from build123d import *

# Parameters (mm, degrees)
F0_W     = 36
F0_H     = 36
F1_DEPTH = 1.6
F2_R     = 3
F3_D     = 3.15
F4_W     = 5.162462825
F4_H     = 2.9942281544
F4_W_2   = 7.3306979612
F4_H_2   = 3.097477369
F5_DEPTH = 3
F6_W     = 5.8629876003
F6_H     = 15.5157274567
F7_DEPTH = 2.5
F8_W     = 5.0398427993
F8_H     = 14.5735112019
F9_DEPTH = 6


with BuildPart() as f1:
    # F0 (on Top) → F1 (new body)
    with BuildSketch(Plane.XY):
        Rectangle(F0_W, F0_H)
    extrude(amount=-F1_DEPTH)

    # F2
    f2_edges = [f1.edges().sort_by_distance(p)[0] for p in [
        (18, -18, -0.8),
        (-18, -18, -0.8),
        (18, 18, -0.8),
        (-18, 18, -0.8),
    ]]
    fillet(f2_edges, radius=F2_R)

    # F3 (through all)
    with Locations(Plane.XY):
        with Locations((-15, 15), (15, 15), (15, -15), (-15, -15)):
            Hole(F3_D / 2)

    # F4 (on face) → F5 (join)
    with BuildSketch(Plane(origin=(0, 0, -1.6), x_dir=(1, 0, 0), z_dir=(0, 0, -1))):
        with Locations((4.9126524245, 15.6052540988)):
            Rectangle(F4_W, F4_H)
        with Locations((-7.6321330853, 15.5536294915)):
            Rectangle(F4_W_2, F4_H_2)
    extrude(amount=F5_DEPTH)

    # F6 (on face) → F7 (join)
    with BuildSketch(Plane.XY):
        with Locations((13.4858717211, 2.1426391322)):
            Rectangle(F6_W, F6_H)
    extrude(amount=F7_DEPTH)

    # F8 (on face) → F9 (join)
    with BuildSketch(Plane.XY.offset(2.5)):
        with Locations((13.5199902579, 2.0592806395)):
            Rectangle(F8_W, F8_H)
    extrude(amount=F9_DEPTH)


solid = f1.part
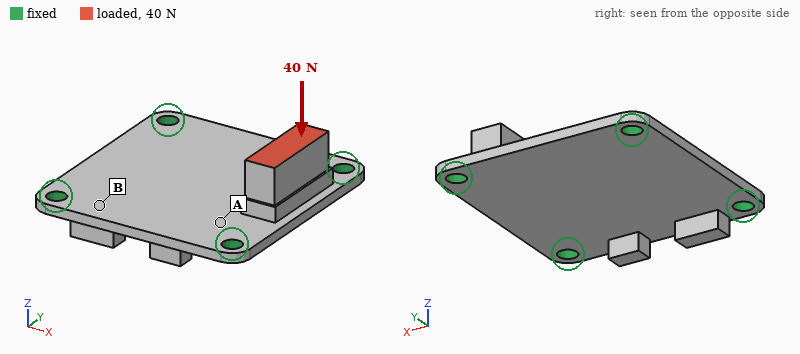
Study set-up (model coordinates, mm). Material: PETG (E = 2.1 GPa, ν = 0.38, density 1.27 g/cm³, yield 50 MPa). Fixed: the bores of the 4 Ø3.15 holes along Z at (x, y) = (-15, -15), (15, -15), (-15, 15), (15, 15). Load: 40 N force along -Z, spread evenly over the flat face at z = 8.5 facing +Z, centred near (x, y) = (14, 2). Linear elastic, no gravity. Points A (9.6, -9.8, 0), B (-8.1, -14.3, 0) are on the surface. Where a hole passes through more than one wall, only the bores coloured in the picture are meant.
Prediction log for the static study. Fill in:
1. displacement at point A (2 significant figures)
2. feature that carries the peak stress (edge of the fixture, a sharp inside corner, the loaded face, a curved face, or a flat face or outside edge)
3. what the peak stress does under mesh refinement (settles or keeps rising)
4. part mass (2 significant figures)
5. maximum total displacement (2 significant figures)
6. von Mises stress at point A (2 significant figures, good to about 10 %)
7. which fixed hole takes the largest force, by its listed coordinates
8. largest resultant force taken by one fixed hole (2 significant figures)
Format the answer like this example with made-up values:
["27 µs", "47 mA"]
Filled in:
["0.076 mm", "edge of the fixture", "keeps rising", "3.5 g", "0.16 mm", "3.5 MPa", "(15, 15)", "24 N"]
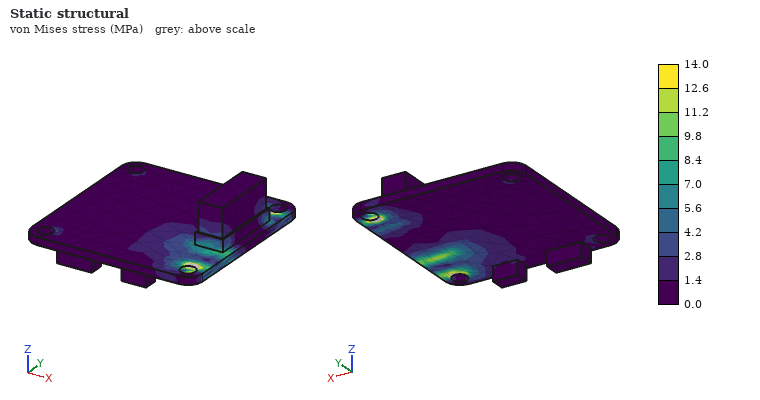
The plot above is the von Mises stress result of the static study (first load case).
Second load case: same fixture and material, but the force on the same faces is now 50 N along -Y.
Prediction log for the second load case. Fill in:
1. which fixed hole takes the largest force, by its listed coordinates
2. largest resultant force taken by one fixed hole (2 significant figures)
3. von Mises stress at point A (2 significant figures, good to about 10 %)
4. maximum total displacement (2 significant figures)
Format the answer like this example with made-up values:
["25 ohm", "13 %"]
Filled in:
["(15, 15)", "31 N", "4.7 MPa", "0.20 mm"]
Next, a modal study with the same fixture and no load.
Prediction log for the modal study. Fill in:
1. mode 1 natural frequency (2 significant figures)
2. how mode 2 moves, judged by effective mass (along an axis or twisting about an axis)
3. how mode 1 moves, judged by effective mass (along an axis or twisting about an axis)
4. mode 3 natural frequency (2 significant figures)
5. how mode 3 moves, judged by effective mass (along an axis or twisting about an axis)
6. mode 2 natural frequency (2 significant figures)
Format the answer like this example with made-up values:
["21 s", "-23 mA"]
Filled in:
["1700 Hz", "along Z", "along Z", "2900 Hz", "twisting about X", "2400 Hz"]
